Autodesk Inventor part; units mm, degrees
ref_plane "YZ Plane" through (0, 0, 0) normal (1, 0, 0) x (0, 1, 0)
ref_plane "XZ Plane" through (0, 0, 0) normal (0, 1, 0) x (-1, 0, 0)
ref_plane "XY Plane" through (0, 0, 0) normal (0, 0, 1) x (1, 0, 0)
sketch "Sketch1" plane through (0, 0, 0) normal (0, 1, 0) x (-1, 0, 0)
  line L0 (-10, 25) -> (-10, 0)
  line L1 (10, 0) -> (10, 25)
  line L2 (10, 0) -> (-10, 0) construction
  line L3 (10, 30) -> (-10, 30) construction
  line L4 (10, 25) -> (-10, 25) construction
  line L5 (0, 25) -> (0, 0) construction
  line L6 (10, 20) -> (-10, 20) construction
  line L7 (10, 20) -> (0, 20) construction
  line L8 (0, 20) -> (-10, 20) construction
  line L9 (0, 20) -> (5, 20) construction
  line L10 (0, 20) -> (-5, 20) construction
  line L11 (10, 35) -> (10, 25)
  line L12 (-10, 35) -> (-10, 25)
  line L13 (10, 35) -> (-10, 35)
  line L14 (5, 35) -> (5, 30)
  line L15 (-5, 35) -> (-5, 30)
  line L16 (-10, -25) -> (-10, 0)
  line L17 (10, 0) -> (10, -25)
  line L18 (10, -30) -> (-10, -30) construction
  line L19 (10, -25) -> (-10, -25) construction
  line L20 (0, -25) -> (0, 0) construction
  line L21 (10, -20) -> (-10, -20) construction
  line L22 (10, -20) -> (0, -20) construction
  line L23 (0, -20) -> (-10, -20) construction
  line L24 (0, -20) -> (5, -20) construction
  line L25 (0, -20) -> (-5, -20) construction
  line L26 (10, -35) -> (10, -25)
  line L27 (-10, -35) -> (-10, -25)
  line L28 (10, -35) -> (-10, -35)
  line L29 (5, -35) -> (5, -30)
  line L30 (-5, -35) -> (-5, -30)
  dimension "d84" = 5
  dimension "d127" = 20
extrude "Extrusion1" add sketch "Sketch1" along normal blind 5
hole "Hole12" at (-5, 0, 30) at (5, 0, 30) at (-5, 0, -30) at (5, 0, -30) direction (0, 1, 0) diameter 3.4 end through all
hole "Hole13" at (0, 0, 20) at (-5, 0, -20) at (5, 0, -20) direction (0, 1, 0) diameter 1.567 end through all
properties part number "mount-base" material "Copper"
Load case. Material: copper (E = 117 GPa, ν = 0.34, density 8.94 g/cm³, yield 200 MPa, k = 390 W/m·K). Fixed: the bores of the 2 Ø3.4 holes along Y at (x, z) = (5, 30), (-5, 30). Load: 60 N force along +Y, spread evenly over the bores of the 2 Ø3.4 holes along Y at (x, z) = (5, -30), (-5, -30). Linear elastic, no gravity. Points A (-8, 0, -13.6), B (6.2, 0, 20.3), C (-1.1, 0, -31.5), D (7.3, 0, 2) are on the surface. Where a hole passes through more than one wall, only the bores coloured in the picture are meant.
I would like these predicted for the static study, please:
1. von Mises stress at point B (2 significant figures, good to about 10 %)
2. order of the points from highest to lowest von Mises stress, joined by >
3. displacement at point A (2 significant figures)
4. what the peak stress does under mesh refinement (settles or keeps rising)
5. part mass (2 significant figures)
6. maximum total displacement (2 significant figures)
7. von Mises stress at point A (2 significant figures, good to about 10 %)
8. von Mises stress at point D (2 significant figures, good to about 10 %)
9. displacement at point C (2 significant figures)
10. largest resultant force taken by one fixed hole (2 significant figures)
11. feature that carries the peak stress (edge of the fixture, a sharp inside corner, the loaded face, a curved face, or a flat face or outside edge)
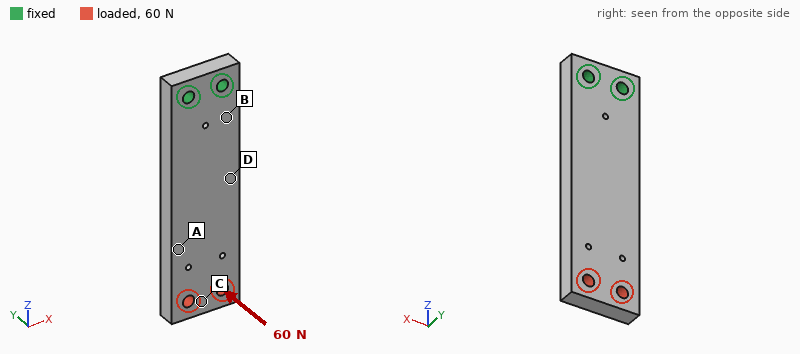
36 MPa
B > D > A > C
0.10 mm
keeps rising
61 g
0.19 mm
12 MPa
23 MPa
0.18 mm
30 N
edge of the fixture
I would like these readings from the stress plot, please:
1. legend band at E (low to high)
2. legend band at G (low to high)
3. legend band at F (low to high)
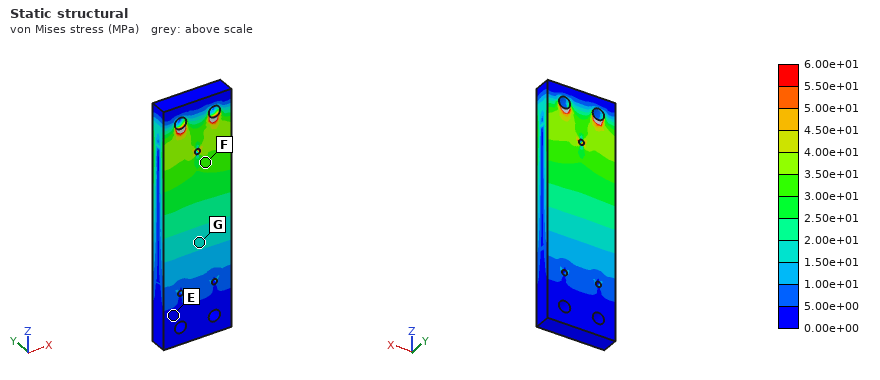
0.00e+00 to 5.00e+00 MPa
1.50e+01 to 2.00e+01 MPa
3.00e+01 to 3.50e+01 MPa
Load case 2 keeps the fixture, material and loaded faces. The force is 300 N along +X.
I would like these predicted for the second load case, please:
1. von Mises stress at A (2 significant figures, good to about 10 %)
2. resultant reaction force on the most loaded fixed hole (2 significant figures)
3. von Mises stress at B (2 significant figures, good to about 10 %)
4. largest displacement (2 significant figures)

12 MPa
1.5 kN
30 MPa
73 µm
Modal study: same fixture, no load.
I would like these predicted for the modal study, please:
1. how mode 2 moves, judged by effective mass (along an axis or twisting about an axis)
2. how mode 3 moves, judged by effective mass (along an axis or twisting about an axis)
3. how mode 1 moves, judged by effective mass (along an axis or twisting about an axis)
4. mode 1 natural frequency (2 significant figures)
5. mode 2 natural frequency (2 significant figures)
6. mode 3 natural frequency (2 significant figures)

along X
twisting about Z
along Y
720 Hz
2500 Hz
4100 Hz
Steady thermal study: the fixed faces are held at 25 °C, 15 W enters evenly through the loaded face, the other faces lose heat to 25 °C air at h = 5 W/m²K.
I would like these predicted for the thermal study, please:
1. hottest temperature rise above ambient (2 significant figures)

24 K
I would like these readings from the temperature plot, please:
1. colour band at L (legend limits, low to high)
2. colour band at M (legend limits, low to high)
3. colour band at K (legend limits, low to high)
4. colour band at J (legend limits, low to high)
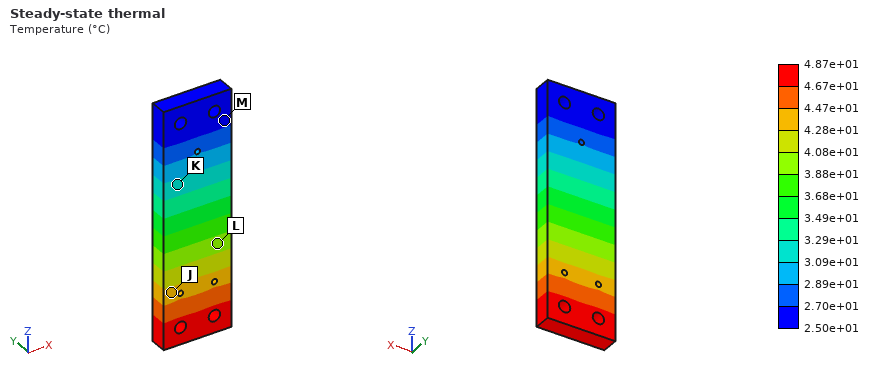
3.88e+01 to 4.08e+01 °C
2.50e+01 to 2.70e+01 °C
3.09e+01 to 3.29e+01 °C
4.28e+01 to 4.47e+01 °C
